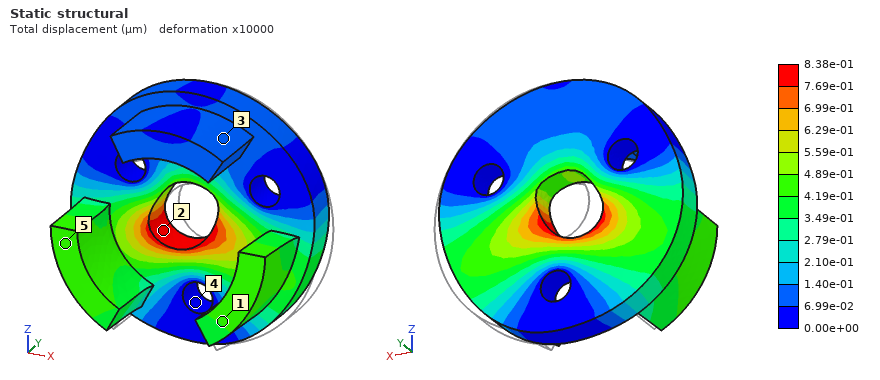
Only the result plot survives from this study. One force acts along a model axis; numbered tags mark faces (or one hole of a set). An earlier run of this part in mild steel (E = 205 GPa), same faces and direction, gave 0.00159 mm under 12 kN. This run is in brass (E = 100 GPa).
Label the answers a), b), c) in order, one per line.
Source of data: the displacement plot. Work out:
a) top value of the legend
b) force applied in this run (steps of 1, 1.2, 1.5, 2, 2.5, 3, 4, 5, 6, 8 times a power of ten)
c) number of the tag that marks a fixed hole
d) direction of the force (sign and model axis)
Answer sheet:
a) 8.38e-01 µm
b) 3 kN
c) 4
d) -X
